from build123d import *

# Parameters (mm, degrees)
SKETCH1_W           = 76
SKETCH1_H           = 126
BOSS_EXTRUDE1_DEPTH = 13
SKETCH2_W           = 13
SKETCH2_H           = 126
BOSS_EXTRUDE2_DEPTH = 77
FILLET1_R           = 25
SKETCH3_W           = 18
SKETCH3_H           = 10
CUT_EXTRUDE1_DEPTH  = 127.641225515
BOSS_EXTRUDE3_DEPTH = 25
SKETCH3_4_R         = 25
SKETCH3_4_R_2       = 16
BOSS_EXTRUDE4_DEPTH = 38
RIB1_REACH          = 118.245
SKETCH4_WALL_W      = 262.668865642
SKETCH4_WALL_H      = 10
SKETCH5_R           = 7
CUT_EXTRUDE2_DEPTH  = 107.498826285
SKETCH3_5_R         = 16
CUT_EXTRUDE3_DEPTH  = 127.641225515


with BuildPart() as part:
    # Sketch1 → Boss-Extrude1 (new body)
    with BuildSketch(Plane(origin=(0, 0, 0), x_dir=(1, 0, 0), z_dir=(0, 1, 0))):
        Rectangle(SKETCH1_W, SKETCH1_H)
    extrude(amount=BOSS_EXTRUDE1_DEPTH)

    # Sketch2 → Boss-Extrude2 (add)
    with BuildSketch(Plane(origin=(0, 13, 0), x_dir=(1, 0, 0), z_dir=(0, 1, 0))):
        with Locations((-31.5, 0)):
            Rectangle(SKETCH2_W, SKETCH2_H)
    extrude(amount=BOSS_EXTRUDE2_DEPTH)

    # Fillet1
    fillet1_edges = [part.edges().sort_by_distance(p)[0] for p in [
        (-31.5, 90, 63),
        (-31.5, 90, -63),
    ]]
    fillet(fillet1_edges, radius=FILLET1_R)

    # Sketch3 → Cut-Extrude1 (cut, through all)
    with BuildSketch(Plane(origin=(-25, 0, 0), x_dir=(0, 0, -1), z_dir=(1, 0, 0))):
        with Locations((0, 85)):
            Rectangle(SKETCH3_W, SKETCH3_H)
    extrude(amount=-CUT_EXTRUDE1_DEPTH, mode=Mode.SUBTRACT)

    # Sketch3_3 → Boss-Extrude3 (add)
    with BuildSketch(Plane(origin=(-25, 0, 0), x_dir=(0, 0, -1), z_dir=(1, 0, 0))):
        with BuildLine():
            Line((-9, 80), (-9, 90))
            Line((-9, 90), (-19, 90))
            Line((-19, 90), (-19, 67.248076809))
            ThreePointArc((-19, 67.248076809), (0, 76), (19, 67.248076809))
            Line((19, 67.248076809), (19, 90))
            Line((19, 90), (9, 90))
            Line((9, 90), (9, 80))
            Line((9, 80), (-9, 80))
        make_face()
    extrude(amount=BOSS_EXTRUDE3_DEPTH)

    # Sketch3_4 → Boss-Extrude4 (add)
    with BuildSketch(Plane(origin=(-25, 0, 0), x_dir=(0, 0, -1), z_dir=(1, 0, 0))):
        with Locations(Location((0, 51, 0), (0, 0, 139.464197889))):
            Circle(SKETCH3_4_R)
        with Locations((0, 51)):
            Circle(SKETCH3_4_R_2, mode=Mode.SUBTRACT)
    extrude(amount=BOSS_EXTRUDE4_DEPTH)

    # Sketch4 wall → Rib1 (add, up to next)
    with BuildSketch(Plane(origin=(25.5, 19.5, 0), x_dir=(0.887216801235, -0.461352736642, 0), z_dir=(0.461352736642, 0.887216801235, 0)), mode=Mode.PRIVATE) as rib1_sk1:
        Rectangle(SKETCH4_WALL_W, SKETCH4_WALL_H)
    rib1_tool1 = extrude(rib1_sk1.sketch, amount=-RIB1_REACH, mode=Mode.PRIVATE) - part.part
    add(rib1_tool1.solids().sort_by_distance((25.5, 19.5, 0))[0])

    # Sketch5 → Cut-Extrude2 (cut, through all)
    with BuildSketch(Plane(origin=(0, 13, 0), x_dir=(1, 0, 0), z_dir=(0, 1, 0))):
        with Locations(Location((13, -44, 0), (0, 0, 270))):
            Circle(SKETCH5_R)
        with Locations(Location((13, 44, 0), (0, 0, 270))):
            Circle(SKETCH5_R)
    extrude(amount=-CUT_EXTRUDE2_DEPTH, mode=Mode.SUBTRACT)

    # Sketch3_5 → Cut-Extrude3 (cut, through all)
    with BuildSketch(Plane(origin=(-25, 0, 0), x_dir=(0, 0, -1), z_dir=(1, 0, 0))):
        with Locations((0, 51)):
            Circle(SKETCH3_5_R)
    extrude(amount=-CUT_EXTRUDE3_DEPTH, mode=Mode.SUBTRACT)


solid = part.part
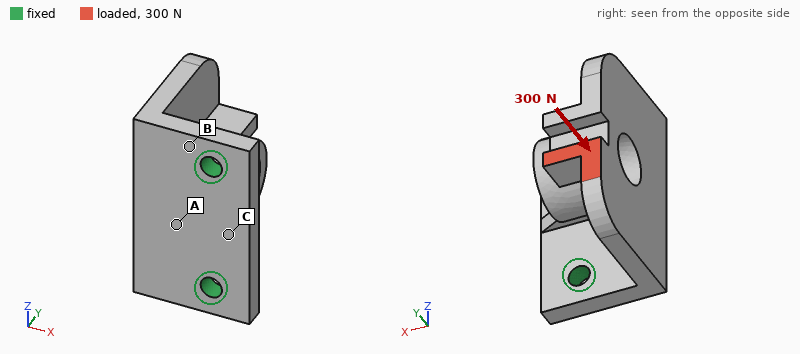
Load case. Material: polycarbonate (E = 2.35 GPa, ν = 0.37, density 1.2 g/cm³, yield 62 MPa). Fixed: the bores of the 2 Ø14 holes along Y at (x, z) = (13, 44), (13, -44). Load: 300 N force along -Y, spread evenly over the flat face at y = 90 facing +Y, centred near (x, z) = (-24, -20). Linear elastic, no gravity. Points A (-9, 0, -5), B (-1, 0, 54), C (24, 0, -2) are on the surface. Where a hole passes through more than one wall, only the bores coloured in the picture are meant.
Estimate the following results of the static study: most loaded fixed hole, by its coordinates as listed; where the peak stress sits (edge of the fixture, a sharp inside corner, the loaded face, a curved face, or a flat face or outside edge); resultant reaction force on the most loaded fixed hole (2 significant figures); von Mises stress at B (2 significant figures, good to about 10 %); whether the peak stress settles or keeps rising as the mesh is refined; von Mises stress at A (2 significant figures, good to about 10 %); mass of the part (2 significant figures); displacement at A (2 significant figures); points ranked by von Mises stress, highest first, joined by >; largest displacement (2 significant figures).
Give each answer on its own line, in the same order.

(13, -44)
edge of the fixture
220 N
1.5 MPa
keeps rising
0.82 MPa
350 g
0.067 mm
B > A > C
0.29 mm
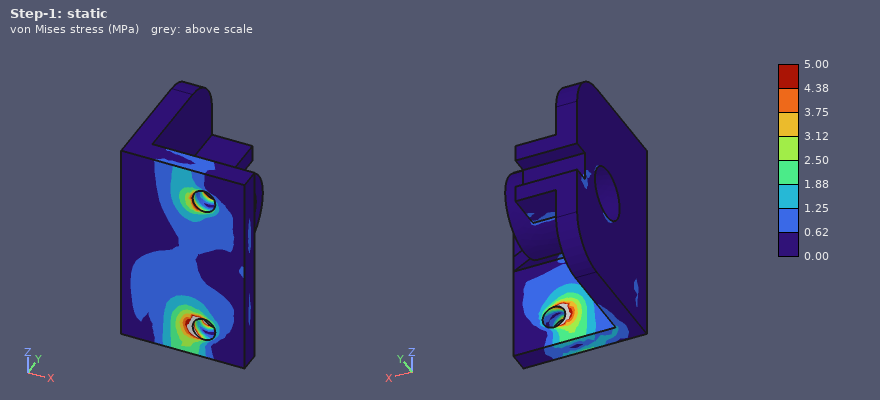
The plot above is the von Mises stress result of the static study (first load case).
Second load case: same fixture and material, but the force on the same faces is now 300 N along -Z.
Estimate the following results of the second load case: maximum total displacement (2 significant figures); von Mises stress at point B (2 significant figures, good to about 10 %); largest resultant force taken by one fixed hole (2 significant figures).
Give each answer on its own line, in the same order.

0.32 mm
2.7 MPa
340 N
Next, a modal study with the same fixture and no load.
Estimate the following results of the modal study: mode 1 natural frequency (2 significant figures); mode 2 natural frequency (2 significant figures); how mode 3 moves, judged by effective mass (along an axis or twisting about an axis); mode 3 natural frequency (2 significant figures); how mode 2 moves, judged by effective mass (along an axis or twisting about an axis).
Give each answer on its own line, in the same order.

310 Hz
520 Hz
along Y
910 Hz
along Z
